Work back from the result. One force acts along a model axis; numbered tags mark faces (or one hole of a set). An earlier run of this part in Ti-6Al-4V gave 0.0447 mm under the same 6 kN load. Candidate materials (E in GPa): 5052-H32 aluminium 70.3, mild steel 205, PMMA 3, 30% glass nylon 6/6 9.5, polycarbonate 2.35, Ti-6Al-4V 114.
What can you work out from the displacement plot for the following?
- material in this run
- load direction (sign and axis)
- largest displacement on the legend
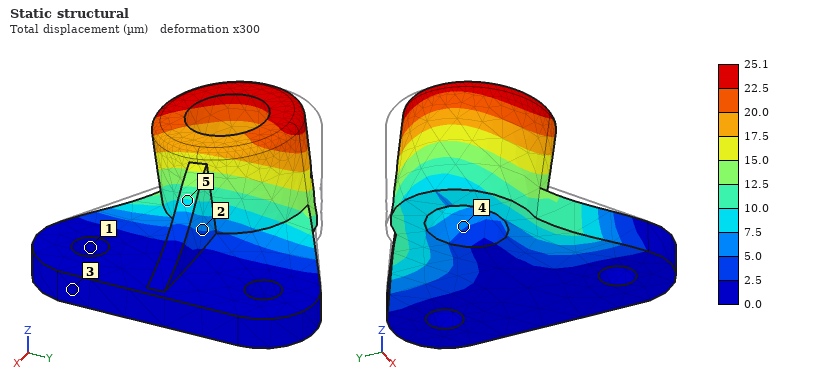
mild steel
-Y
25.1 µm
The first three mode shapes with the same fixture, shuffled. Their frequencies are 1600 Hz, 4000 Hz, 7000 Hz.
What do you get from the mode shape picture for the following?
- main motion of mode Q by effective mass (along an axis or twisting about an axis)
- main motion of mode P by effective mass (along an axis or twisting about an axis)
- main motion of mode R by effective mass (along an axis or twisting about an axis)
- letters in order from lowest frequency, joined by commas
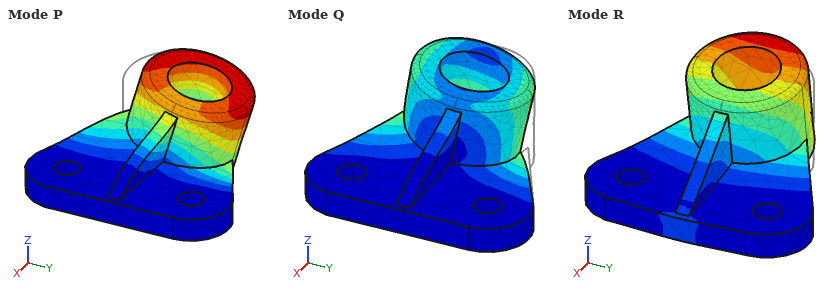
along Y
along Y
along Z
R, P, Q
